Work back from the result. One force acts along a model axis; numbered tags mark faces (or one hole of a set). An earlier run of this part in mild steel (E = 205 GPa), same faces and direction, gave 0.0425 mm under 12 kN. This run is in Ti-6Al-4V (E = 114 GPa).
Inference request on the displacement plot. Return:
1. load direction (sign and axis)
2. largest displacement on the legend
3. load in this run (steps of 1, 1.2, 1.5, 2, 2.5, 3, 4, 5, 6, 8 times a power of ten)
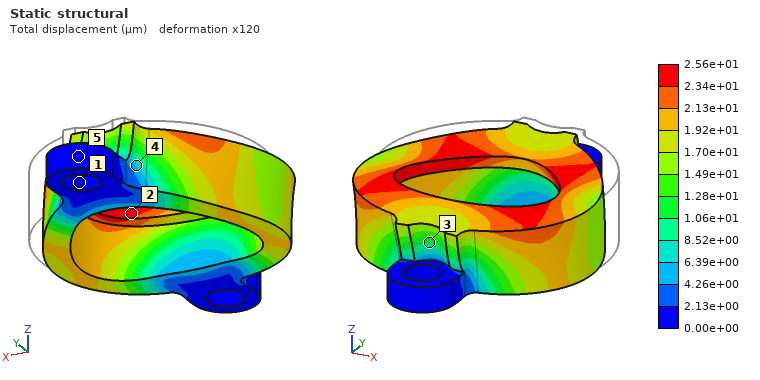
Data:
-Y
2.56e+01 µm
4 kN
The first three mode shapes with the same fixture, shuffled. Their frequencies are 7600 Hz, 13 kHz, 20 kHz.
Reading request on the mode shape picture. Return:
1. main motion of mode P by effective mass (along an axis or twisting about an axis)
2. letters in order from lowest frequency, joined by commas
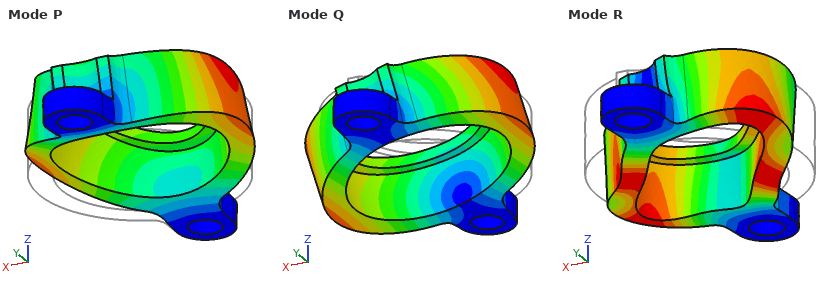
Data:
along Z
Q, P, R
